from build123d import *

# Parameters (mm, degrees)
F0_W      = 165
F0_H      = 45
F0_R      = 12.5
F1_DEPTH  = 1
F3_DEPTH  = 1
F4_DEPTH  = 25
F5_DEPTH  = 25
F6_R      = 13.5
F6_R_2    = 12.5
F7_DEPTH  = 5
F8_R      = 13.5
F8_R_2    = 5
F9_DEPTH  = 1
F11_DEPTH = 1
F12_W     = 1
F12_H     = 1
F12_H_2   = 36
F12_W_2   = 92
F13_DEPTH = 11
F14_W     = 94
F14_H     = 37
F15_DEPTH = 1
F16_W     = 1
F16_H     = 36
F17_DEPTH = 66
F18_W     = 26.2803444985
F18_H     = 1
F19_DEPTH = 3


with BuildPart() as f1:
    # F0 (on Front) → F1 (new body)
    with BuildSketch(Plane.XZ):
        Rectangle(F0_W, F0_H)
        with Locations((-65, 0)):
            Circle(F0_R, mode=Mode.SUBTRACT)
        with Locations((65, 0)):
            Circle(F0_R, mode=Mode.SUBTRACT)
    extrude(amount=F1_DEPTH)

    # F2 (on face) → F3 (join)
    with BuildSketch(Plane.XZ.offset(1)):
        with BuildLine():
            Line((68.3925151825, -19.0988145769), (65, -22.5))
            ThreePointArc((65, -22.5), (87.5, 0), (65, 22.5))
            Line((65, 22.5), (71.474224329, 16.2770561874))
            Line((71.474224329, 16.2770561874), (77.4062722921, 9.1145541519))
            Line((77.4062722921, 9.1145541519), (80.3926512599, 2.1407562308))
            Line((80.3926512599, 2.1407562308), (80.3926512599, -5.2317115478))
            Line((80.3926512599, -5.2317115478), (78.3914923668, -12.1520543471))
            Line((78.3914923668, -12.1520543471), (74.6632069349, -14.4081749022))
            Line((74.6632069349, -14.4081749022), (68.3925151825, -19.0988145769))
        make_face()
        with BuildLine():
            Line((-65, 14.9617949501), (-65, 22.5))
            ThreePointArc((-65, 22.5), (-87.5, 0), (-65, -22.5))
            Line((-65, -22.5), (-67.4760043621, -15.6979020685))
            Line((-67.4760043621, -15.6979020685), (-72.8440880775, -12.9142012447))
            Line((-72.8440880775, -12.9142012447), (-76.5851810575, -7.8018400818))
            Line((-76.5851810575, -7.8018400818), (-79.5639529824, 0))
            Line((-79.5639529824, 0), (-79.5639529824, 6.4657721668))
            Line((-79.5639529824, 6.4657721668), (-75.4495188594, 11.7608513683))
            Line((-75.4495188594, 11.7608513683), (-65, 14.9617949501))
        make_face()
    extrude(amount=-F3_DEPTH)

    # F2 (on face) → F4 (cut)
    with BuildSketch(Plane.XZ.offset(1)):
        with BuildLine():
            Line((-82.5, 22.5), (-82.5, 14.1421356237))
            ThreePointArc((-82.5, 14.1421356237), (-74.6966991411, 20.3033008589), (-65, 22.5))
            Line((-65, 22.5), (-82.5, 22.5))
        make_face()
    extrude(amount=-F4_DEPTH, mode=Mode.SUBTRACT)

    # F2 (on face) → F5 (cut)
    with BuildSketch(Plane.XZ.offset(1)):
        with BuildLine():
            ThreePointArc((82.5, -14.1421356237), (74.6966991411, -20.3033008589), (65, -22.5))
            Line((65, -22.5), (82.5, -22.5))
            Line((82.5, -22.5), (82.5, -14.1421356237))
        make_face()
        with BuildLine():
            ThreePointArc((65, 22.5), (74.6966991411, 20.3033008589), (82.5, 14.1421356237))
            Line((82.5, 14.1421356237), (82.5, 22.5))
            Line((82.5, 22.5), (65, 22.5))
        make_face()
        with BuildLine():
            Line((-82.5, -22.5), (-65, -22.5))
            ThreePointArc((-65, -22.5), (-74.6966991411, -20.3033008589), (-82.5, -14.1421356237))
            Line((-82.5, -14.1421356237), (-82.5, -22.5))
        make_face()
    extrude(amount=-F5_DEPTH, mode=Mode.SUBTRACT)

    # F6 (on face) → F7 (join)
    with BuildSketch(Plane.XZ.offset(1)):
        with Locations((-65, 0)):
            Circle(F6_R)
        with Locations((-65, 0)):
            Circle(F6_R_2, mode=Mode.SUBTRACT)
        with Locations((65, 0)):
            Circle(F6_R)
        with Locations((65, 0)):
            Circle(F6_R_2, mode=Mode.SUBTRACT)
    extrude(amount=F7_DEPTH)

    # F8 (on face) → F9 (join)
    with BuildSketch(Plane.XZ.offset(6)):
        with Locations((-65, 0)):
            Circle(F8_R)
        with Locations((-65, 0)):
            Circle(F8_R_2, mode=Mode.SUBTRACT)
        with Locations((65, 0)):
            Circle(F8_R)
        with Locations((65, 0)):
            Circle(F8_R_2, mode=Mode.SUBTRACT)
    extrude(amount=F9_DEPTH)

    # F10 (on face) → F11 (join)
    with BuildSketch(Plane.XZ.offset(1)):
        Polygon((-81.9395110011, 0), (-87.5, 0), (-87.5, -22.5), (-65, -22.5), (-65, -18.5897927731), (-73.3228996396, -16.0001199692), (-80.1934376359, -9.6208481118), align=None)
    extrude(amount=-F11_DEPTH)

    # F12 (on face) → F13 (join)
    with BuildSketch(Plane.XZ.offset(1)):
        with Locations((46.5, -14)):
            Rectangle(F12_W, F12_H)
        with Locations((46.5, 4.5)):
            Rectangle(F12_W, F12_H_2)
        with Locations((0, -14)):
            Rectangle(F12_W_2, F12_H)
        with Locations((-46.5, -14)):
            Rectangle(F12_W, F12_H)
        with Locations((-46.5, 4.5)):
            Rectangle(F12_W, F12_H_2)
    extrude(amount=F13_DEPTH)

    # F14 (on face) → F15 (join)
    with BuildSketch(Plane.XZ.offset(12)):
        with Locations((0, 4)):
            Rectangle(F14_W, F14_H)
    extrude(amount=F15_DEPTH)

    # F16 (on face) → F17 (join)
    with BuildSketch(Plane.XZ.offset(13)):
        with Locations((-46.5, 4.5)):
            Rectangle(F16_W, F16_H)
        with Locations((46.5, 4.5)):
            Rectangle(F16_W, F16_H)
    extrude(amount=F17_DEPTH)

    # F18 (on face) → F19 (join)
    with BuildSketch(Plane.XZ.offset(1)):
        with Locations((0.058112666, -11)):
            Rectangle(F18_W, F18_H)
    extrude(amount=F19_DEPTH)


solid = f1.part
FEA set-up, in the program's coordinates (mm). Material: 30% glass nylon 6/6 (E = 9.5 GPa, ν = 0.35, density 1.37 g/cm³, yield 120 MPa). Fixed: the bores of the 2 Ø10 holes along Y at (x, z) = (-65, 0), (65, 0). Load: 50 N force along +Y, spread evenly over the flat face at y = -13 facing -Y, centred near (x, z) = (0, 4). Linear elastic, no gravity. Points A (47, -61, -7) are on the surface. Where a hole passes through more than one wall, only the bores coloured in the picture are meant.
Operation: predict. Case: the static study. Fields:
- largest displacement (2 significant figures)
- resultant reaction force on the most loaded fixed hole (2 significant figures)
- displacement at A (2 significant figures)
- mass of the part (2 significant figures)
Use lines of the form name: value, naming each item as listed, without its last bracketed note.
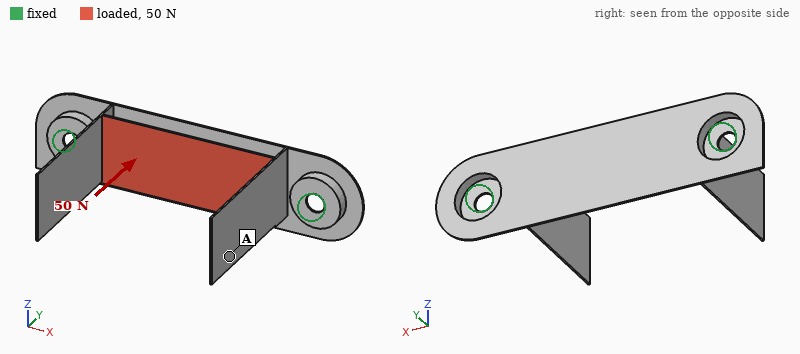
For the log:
largest displacement: 2.2 mm
resultant reaction force on the most loaded fixed hole: 47 N
displacement at A: 0.47 mm
mass of the part: 25 g
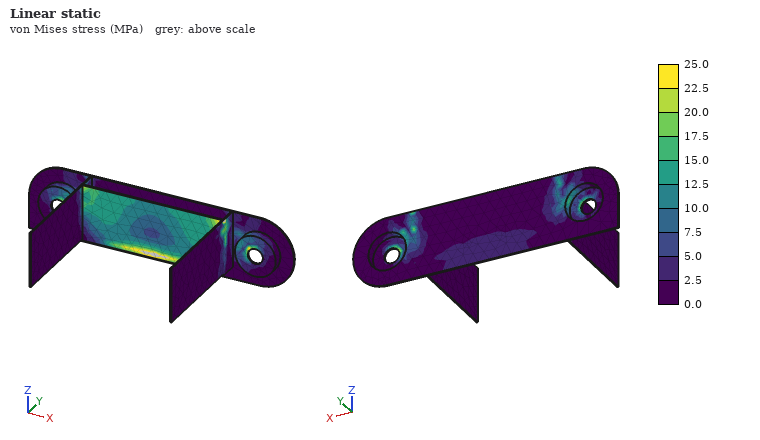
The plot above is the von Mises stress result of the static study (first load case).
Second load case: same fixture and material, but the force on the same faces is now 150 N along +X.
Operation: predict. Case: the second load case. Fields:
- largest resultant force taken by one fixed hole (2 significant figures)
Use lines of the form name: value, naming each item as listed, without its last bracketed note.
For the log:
largest resultant force taken by one fixed hole: 80 N
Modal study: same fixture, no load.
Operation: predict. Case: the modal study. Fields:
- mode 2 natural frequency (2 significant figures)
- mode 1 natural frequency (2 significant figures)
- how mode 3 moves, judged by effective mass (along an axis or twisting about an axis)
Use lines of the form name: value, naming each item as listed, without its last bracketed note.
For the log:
mode 2 natural frequency: 95 Hz
mode 1 natural frequency: 93 Hz
how mode 3 moves, judged by effective mass: along Z
